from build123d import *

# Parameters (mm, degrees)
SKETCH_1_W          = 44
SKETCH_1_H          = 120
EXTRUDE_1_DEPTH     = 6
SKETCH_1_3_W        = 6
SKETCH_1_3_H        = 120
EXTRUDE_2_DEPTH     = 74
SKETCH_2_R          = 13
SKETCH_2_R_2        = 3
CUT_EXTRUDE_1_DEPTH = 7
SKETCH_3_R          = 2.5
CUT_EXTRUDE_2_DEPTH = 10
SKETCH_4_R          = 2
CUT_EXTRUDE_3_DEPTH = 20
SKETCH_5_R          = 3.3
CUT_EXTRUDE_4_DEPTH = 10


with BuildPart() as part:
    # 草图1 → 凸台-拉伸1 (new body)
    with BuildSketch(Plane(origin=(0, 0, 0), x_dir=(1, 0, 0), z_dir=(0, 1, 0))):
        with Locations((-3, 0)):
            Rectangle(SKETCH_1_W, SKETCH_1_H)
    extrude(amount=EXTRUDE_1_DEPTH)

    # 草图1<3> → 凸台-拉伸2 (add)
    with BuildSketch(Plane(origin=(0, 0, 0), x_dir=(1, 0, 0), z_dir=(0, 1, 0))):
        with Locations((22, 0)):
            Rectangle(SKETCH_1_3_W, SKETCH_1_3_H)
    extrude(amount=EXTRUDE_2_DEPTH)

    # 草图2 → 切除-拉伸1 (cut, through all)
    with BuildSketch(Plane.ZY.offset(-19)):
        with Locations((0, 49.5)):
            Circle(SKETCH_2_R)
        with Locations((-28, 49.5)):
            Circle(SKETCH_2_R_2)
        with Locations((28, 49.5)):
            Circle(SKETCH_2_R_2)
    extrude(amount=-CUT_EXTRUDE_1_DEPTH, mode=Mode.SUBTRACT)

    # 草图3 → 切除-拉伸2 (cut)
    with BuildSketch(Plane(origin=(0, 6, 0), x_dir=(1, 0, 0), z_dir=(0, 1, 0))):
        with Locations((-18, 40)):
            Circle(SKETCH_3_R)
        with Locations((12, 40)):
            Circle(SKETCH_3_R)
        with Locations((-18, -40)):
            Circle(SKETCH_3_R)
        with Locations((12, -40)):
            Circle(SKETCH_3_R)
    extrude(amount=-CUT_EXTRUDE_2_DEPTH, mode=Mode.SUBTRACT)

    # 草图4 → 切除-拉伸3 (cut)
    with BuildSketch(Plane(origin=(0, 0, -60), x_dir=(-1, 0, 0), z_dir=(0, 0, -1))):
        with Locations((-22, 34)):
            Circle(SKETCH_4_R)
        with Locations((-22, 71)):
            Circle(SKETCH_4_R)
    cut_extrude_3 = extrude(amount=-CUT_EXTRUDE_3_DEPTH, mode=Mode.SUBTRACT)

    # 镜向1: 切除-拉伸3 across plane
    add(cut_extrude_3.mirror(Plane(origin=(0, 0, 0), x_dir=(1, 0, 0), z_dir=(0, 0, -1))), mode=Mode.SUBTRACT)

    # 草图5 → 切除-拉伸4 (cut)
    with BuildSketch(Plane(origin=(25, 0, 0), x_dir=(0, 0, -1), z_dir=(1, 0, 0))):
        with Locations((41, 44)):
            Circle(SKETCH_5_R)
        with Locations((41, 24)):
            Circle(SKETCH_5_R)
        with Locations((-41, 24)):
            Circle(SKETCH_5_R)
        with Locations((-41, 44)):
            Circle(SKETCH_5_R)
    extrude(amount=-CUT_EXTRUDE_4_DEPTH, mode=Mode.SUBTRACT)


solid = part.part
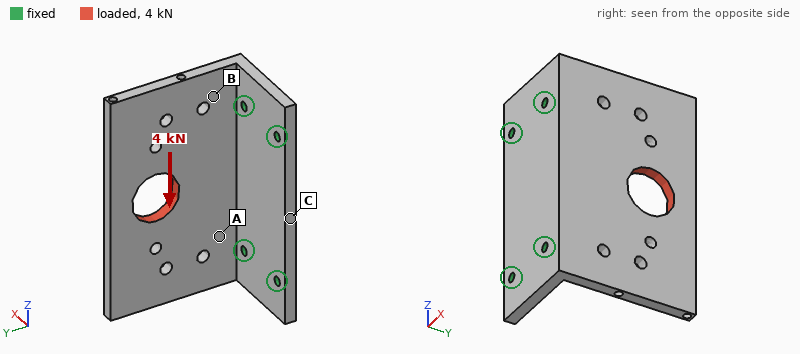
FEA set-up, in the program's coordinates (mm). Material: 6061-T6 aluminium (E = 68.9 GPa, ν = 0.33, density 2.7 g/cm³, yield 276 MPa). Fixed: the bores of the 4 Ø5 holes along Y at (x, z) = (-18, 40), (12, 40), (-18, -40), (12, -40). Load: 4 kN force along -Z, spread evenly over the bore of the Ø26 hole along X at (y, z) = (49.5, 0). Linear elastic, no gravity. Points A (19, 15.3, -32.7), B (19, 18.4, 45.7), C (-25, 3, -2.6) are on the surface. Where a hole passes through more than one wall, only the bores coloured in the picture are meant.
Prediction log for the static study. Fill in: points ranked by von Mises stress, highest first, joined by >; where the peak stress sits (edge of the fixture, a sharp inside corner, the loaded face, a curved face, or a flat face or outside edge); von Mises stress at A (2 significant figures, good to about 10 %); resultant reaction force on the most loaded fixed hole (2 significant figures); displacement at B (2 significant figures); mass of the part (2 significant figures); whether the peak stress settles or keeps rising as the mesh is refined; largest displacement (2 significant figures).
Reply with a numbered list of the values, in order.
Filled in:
1. A > B > C
2. edge of the fixture
3. 28 MPa
4. 3.0 kN
5. 0.040 mm
6. 210 g
7. keeps rising
8. 0.12 mm
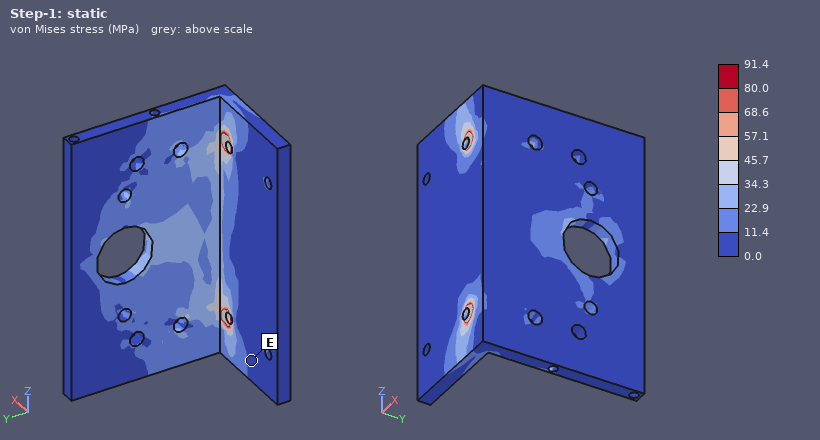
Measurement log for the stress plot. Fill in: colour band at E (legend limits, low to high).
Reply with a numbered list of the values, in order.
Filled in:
1. 0.0 to 11.4 MPa
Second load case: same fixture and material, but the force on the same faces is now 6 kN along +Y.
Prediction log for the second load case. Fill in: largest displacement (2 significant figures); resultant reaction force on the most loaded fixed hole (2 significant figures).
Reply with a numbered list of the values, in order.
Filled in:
1. 0.24 mm
2. 3.5 kN
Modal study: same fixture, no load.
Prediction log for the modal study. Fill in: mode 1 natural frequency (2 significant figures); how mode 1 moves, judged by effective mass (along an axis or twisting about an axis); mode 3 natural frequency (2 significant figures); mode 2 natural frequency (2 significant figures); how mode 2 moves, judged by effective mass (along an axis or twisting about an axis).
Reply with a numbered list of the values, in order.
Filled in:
1. 820 Hz
2. along X
3. 3200 Hz
4. 1400 Hz
5. twisting about Y
